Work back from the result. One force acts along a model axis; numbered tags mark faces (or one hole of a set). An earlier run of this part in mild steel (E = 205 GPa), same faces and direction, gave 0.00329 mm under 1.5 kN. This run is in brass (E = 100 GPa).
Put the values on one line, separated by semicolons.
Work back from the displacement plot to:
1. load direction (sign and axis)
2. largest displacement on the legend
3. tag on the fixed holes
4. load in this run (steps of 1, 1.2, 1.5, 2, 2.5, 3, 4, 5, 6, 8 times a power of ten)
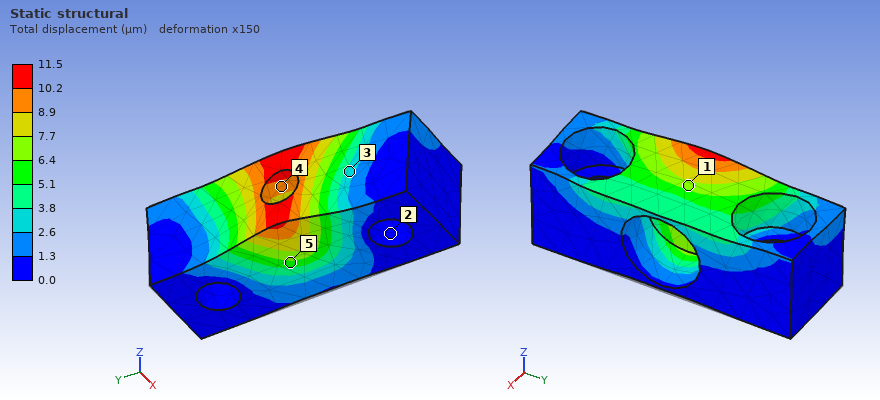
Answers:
+Z; 11.5 µm; 2; 2.5 kN
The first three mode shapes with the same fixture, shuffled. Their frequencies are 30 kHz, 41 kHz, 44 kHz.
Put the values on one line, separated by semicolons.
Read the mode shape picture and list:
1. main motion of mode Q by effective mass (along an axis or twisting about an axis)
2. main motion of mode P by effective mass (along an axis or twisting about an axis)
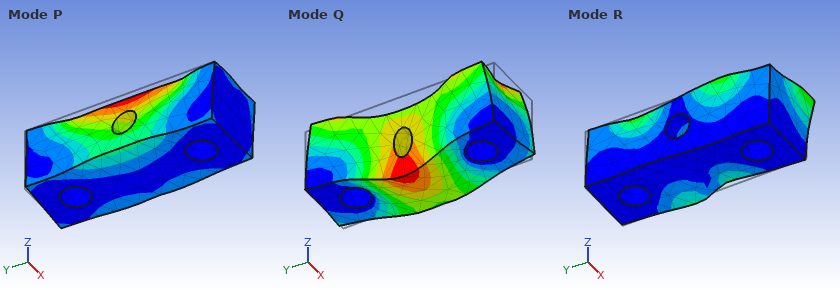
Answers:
along Z; along X
